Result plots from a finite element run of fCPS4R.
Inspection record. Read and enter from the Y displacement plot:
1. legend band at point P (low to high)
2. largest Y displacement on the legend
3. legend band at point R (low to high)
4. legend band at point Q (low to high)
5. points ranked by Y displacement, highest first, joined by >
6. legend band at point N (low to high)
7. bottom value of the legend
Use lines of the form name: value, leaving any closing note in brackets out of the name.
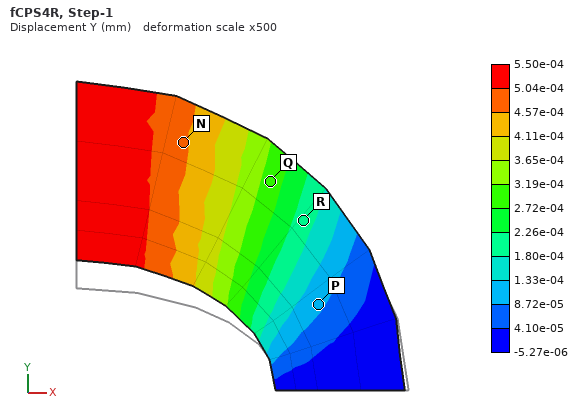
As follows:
legend band at point P: 8.72e-05 to 1.33e-04 mm
largest Y displacement on the legend: 5.50e-04 mm
legend band at point R: 1.80e-04 to 2.26e-04 mm
legend band at point Q: 2.72e-04 to 3.19e-04 mm
points ranked by Y displacement, highest first, joined by >: N > Q > R > P
legend band at point N: 4.57e-04 to 5.04e-04 mm
bottom value of the legend: -5.27e-06 mm
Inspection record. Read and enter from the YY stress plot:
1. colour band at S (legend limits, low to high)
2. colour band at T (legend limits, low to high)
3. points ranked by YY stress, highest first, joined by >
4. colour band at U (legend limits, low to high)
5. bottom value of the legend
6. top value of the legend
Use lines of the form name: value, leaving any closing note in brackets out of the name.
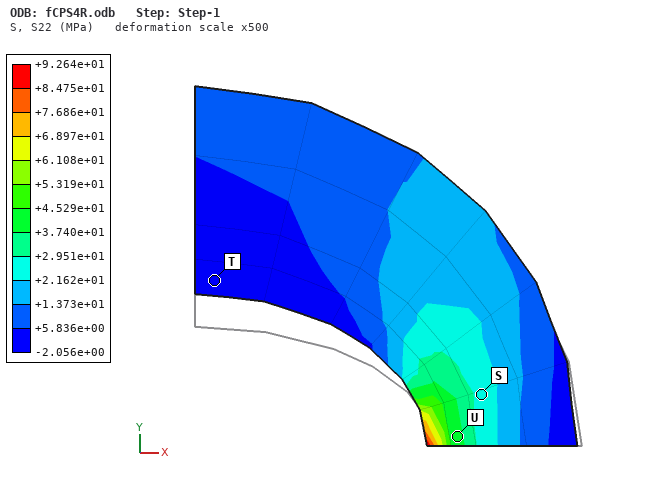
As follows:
colour band at S: +2.162e+01 to +2.951e+01 MPa
colour band at T: -2.056e+00 to +5.836e+00 MPa
points ranked by YY stress, highest first, joined by >: U > S > T
colour band at U: +3.740e+01 to +4.529e+01 MPa
bottom value of the legend: -2.056e+00 MPa
top value of the legend: +9.264e+01 MPa
